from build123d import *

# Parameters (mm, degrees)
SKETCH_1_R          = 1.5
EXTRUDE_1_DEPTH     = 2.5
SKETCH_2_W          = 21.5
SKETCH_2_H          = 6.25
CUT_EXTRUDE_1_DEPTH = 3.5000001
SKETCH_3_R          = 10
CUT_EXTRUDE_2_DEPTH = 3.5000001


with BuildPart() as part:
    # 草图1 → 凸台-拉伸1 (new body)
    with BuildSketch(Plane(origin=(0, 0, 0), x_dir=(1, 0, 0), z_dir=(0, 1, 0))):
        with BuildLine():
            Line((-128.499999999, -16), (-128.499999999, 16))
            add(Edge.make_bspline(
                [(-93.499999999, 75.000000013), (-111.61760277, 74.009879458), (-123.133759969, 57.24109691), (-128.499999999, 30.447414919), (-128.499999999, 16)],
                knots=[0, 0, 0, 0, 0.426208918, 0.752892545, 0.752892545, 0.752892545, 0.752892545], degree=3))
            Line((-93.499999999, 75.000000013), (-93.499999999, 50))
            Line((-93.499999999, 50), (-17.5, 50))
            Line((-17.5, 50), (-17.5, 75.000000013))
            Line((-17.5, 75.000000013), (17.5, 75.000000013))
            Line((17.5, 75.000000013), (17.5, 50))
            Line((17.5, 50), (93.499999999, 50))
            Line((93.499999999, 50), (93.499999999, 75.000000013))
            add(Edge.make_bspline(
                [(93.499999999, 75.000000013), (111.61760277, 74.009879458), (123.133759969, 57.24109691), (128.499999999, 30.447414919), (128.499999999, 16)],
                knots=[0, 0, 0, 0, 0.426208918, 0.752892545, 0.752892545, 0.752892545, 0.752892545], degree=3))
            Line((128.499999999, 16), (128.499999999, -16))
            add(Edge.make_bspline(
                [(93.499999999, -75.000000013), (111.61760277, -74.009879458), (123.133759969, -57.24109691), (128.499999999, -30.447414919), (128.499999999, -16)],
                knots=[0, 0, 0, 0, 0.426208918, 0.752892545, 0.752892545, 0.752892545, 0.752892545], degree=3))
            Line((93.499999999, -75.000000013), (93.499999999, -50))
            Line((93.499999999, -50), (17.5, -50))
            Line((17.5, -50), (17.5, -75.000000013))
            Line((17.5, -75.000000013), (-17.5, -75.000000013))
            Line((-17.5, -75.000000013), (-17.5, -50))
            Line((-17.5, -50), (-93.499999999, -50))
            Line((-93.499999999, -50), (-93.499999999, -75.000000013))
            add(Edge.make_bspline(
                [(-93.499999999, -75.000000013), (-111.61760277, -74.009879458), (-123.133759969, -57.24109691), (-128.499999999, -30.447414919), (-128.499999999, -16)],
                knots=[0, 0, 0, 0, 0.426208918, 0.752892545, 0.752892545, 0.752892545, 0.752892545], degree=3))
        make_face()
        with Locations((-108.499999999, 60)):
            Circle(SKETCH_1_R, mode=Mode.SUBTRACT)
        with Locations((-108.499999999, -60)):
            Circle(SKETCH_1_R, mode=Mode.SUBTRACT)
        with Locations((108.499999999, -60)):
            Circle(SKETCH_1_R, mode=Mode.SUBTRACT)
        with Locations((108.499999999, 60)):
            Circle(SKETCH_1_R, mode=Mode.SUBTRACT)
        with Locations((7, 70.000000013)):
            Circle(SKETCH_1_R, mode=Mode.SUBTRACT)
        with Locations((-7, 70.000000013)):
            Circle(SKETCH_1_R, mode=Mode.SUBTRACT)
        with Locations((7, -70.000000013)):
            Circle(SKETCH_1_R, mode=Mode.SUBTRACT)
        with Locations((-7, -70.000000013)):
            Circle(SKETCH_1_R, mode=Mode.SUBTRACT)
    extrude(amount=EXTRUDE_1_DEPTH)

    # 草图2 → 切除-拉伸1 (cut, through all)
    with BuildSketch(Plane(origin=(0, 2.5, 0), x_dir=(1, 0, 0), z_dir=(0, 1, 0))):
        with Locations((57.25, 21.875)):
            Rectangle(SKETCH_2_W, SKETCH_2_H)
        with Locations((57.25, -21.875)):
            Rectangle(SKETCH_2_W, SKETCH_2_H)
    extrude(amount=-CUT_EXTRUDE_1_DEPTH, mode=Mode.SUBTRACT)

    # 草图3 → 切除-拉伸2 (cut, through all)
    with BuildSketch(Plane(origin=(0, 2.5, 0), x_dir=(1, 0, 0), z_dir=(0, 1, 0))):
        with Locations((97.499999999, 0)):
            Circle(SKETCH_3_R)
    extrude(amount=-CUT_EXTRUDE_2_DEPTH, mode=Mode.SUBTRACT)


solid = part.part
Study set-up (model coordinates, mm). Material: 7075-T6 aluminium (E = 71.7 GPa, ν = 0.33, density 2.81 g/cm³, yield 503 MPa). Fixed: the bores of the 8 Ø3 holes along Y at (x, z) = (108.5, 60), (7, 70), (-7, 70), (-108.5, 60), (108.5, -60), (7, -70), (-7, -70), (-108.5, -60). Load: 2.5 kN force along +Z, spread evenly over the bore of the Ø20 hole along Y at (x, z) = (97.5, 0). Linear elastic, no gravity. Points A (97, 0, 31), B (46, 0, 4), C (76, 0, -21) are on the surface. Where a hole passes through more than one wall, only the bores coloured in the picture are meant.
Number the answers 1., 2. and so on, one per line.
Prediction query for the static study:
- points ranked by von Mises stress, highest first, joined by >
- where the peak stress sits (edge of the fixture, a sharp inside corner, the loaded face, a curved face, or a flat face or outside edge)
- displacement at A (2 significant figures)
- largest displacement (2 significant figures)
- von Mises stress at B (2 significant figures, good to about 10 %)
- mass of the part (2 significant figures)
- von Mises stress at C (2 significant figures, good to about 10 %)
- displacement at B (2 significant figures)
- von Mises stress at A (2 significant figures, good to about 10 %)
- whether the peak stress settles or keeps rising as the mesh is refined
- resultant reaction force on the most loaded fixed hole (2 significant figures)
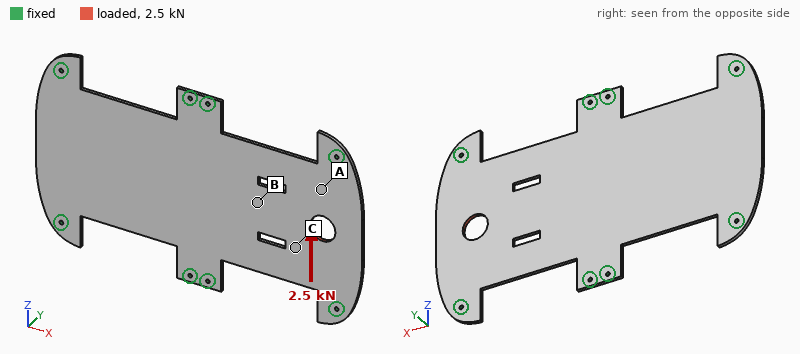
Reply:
1. A > C > B
2. edge of the fixture
3. 9.4 µm
4. 14 µm
5. 2.6 MPa
6. 200 g
7. 6.4 MPa
8. 5.0 µm
9. 13 MPa
10. keeps rising
11. 1.1 kN
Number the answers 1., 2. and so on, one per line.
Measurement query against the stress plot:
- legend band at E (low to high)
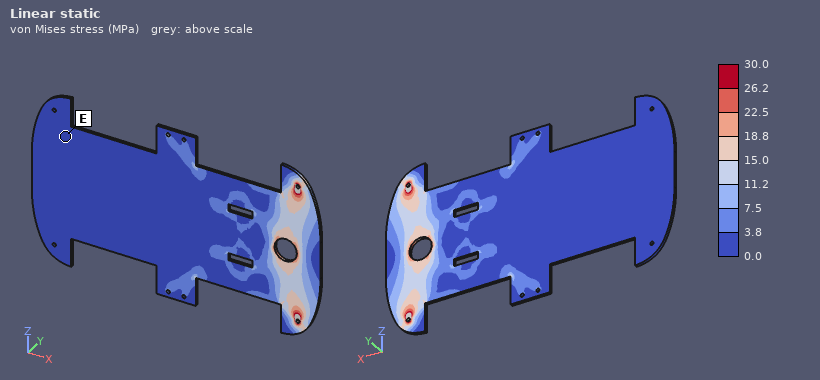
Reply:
1. 0.0 to 3.8 MPa
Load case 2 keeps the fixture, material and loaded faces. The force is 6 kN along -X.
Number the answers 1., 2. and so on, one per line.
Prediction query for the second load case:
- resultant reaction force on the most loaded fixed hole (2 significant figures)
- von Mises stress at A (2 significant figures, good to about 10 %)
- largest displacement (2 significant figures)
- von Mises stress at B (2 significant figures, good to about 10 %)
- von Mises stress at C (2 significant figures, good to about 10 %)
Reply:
1. 1.3 kN
2. 22 MPa
3. 71 µm
4. 18 MPa
5. 38 MPa
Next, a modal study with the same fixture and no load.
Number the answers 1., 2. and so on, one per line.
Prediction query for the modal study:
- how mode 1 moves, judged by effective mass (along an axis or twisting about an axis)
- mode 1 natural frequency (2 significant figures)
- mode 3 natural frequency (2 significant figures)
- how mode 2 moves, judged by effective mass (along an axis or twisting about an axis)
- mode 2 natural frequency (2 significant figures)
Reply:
1. along Y
2. 520 Hz
3. 880 Hz
4. twisting about Z
5. 630 Hz
